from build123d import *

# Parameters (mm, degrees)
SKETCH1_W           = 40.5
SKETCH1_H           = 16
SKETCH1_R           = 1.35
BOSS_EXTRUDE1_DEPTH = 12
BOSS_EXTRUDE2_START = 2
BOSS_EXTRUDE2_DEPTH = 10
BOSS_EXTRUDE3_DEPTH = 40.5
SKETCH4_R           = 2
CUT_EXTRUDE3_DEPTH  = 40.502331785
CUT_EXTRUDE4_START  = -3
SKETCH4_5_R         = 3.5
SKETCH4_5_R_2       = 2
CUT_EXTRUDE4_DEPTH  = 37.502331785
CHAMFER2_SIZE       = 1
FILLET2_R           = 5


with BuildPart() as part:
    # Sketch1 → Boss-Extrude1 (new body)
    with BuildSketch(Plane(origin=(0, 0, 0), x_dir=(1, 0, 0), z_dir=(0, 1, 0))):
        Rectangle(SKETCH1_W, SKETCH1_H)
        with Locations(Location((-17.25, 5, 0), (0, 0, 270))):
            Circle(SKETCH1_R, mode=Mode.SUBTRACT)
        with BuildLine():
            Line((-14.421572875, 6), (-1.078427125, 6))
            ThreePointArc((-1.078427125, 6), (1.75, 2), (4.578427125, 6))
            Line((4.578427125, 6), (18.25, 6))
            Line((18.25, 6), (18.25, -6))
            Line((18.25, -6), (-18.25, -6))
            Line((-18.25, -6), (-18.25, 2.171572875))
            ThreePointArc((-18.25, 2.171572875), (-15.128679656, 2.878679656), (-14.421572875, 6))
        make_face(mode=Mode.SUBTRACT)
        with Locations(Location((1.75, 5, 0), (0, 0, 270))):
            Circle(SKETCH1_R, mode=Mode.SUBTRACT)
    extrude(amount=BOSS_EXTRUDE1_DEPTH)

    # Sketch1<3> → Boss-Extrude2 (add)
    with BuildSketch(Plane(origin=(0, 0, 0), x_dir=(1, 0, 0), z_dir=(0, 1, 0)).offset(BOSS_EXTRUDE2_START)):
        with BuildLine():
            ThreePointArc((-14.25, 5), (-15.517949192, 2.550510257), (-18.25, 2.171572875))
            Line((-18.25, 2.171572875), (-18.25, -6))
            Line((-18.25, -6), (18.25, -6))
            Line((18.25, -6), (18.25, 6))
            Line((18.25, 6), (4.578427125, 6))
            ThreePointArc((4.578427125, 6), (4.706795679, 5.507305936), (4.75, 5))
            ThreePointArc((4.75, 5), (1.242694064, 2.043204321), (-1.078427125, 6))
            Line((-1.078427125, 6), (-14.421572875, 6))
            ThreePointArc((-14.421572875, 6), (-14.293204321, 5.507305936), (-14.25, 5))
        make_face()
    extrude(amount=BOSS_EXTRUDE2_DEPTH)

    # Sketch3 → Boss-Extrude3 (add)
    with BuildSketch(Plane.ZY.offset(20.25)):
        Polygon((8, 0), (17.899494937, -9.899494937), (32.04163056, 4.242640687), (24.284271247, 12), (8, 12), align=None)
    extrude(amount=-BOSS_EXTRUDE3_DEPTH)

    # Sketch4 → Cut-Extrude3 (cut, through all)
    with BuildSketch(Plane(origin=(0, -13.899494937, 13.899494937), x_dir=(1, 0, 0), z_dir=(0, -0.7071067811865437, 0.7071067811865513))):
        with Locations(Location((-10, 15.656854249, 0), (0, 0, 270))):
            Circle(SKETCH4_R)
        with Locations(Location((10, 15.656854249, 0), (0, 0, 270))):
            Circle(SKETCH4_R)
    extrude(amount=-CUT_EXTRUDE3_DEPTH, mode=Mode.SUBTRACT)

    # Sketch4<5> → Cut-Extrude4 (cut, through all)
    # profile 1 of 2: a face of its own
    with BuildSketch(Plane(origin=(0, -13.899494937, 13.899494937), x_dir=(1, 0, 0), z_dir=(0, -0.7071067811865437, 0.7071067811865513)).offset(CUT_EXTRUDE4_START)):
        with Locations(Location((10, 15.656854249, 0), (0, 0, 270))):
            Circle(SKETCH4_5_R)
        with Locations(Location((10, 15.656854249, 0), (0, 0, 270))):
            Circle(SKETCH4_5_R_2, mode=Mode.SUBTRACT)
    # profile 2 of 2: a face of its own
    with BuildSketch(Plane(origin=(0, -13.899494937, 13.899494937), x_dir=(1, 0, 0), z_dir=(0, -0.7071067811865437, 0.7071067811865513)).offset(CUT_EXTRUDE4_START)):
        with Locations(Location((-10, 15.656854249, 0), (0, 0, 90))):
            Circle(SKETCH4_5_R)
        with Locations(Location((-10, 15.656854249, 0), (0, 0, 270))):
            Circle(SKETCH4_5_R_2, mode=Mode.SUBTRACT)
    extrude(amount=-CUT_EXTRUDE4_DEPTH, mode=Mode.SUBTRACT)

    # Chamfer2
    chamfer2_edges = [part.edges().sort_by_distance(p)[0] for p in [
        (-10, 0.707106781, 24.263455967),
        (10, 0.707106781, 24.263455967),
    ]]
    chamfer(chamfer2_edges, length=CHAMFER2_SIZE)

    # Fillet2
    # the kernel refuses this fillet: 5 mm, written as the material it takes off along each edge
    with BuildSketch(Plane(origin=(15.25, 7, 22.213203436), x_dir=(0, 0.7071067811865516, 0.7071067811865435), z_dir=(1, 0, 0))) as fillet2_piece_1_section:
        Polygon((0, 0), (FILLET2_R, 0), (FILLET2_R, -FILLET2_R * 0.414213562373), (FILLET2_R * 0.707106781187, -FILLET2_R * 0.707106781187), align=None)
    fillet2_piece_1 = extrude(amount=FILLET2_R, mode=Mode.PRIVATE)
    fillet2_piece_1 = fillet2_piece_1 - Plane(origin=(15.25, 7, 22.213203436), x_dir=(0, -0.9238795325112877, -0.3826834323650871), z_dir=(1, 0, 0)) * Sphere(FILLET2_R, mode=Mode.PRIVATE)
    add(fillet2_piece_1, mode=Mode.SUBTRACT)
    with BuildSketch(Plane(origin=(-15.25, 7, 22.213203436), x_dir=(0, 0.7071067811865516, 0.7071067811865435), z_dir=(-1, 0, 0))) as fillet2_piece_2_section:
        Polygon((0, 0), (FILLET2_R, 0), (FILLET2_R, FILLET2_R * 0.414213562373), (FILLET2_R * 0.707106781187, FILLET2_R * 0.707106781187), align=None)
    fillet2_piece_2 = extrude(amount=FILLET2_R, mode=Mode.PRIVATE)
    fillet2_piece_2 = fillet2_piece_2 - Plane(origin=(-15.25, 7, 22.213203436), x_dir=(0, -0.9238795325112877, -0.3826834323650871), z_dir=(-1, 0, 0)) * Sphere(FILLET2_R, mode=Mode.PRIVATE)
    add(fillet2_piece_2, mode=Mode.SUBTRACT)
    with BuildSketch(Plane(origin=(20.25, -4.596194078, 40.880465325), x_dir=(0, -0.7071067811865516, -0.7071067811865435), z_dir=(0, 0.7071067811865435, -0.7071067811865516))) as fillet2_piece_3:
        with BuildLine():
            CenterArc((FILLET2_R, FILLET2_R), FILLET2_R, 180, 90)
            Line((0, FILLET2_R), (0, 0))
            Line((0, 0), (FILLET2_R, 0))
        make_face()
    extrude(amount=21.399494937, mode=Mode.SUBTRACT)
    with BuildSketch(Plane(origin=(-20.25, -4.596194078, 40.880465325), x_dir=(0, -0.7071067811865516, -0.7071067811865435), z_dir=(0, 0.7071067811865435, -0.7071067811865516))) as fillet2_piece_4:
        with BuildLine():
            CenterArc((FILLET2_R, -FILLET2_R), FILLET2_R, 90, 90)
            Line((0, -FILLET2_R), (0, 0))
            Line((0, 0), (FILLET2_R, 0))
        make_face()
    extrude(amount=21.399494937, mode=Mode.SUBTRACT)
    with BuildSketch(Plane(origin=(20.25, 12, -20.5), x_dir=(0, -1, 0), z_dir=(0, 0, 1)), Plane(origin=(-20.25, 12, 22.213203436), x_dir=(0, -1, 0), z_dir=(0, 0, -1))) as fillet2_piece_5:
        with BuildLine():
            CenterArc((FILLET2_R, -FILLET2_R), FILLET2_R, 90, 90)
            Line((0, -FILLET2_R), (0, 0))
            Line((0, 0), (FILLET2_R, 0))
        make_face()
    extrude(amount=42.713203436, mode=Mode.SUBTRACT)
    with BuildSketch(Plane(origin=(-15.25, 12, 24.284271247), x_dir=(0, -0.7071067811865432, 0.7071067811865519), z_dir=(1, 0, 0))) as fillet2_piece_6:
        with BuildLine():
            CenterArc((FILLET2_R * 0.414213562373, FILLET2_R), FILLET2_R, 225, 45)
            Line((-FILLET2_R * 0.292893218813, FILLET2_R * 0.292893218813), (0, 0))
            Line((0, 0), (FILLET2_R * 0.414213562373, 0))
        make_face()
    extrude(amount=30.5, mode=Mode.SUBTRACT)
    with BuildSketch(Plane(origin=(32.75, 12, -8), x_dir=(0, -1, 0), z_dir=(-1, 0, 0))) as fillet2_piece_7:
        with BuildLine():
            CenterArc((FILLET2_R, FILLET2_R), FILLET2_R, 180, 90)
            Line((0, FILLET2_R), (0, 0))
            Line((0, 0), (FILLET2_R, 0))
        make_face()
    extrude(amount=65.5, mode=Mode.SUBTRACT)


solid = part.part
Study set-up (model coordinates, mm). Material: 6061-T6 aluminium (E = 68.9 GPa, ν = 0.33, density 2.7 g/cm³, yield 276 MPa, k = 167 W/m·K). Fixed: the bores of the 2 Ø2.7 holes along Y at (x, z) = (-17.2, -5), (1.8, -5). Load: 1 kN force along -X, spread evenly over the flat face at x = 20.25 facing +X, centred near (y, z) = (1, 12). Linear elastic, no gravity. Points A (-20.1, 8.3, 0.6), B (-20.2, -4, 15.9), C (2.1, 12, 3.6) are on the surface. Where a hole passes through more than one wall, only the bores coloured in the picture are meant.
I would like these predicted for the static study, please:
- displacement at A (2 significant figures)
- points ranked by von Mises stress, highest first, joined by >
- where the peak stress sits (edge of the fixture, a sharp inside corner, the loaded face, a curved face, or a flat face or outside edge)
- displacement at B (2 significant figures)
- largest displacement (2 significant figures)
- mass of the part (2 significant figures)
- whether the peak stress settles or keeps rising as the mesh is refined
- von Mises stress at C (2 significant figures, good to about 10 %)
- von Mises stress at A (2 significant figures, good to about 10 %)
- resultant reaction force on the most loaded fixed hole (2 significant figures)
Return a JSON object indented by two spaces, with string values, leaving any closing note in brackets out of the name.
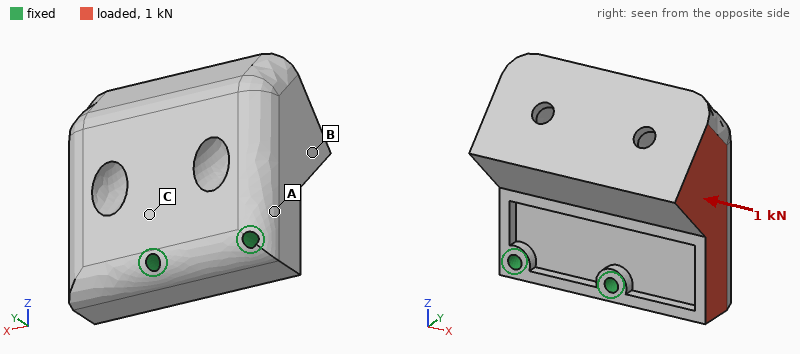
{
  "displacement at A": "2.1 µm",
  "points ranked by von Mises stress, highest first, joined by >": "A > C > B",
  "where the peak stress sits": "edge of the fixture",
  "displacement at B": "7.8 µm",
  "largest displacement": "12 µm",
  "mass of the part": "51 g",
  "whether the peak stress settles or keeps rising as the mesh is refined": "keeps rising",
  "von Mises stress at C": "4.6 MPa",
  "von Mises stress at A": "13 MPa",
  "resultant reaction force on the most loaded fixed hole": "990 N"
}
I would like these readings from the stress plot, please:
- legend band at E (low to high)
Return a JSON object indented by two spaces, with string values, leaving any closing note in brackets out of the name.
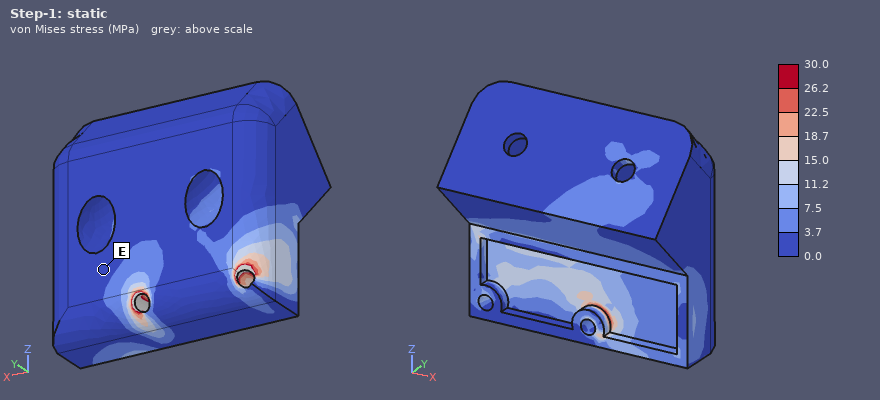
{
  "legend band at E": "0.0 to 3.7 MPa"
}
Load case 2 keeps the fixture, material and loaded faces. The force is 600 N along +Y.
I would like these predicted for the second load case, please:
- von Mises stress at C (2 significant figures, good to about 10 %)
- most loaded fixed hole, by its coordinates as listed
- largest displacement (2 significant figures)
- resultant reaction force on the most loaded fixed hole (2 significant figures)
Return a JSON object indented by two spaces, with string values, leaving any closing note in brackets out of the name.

{
  "von Mises stress at C": "15 MPa",
  "most loaded fixed hole, by its coordinates as listed": "(1.8, -5)",
  "largest displacement": "40 µm",
  "resultant reaction force on the most loaded fixed hole": "880 N"
}
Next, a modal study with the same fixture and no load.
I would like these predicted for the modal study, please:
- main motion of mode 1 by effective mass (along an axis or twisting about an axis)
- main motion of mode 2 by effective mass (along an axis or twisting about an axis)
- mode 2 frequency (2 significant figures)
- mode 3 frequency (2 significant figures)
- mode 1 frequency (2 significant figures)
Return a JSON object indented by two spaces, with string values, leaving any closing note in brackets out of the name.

{
  "main motion of mode 1 by effective mass": "along Y",
  "main motion of mode 2 by effective mass": "along X",
  "mode 2 frequency": "8000 Hz",
  "mode 3 frequency": "9600 Hz",
  "mode 1 frequency": "4200 Hz"
}
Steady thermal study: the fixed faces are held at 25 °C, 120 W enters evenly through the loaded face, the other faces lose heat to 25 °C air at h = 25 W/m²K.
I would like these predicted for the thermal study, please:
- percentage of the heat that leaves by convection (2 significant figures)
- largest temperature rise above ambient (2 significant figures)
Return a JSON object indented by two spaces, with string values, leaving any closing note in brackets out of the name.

{
  "percentage of the heat that leaves by convection": "3.7 %",
  "largest temperature rise above ambient": "69 K"
}
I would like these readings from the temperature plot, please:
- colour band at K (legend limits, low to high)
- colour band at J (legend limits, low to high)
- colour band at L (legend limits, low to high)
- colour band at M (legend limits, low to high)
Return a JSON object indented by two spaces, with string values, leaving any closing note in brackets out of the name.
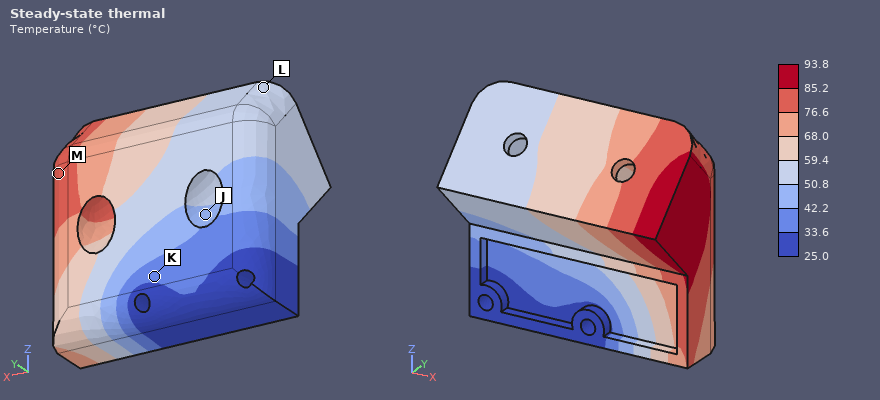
{
  "colour band at K": "33.6 to 42.2 °C",
  "colour band at J": "42.2 to 50.8 °C",
  "colour band at L": "50.8 to 59.4 °C",
  "colour band at M": "76.6 to 85.2 °C"
}
